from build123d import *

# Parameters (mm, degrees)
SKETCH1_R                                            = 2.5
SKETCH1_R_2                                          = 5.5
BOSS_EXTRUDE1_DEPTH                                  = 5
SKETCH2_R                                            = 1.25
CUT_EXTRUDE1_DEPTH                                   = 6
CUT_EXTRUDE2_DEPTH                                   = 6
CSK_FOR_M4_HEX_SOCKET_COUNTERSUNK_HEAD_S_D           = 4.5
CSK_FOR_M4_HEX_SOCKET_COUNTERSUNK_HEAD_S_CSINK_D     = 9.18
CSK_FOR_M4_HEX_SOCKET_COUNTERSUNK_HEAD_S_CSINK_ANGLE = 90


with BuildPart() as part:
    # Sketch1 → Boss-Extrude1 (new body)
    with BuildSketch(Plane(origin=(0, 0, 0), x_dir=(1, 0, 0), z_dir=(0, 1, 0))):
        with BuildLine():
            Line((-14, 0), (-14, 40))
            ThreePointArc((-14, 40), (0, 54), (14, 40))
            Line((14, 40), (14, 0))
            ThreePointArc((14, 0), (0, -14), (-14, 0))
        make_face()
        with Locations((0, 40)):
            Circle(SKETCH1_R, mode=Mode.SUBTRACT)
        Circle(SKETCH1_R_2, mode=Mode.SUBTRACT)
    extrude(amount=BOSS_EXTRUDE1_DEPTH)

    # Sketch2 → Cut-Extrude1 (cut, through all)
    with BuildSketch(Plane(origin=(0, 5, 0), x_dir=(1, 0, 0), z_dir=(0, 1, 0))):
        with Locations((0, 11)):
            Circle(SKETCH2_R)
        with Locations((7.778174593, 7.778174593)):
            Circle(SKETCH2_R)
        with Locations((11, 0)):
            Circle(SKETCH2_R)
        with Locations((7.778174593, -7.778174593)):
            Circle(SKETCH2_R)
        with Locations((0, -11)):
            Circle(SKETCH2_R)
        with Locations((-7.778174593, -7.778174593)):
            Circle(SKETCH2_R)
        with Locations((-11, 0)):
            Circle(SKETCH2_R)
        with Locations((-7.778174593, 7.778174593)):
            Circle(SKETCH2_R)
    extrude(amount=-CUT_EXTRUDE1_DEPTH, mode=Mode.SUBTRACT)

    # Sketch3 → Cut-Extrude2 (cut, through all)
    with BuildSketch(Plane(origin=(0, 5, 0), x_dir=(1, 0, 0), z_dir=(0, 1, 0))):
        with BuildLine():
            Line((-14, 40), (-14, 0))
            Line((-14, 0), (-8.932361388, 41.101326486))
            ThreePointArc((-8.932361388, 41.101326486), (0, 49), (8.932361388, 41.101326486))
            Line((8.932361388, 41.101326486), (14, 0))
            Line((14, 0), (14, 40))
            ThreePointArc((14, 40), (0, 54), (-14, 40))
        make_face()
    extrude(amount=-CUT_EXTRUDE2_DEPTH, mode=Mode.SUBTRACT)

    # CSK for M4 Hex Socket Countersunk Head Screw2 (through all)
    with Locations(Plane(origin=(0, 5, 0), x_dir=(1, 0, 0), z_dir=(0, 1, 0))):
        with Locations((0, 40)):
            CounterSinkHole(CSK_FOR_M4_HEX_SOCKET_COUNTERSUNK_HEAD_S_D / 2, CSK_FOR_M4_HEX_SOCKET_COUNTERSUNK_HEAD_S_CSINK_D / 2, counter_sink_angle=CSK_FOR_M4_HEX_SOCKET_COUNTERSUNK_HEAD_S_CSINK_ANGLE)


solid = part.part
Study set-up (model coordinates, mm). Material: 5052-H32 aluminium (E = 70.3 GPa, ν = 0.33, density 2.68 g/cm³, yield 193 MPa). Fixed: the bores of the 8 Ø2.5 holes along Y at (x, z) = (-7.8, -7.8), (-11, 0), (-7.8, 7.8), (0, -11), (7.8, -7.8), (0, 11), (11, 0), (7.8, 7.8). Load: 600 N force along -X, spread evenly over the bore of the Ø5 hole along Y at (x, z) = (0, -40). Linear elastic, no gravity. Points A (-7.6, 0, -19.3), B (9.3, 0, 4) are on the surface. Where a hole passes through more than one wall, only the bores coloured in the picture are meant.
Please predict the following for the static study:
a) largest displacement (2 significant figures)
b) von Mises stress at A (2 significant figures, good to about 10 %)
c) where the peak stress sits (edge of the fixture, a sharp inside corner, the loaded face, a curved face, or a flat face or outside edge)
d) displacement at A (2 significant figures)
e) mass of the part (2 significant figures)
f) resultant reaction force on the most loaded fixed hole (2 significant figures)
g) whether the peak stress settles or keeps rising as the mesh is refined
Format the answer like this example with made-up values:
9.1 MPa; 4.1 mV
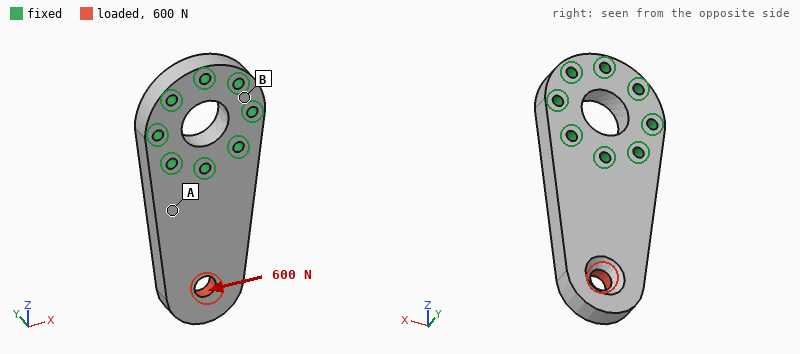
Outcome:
35 µm; 21 MPa; edge of the fixture; 5.9 µm; 16 g; 790 N; keeps rising
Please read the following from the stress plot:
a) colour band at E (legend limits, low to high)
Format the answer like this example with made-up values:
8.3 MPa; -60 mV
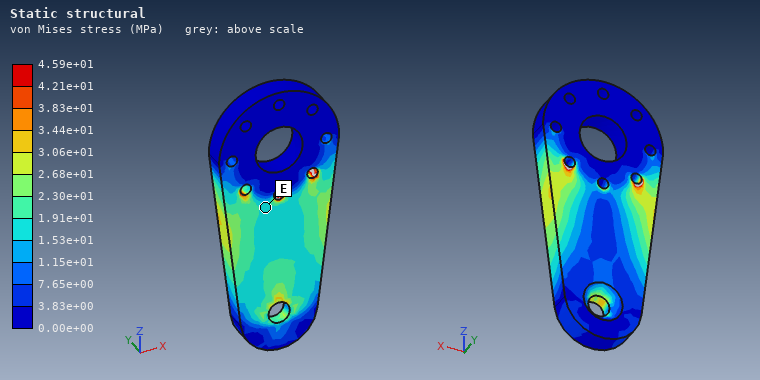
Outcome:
1.53e+01 to 1.91e+01 MPa
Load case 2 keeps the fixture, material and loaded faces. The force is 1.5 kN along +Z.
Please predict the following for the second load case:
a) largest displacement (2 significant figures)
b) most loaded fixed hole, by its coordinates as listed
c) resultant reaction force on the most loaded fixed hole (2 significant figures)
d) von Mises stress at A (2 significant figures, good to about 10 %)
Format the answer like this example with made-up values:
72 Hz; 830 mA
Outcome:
71 µm; (0, -11); 580 N; 28 MPa
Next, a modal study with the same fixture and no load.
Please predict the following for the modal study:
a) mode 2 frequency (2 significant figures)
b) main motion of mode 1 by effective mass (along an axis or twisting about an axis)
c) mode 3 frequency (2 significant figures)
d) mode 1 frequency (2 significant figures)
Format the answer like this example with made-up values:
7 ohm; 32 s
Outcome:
12 kHz; along Y; 12 kHz; 3500 Hz
